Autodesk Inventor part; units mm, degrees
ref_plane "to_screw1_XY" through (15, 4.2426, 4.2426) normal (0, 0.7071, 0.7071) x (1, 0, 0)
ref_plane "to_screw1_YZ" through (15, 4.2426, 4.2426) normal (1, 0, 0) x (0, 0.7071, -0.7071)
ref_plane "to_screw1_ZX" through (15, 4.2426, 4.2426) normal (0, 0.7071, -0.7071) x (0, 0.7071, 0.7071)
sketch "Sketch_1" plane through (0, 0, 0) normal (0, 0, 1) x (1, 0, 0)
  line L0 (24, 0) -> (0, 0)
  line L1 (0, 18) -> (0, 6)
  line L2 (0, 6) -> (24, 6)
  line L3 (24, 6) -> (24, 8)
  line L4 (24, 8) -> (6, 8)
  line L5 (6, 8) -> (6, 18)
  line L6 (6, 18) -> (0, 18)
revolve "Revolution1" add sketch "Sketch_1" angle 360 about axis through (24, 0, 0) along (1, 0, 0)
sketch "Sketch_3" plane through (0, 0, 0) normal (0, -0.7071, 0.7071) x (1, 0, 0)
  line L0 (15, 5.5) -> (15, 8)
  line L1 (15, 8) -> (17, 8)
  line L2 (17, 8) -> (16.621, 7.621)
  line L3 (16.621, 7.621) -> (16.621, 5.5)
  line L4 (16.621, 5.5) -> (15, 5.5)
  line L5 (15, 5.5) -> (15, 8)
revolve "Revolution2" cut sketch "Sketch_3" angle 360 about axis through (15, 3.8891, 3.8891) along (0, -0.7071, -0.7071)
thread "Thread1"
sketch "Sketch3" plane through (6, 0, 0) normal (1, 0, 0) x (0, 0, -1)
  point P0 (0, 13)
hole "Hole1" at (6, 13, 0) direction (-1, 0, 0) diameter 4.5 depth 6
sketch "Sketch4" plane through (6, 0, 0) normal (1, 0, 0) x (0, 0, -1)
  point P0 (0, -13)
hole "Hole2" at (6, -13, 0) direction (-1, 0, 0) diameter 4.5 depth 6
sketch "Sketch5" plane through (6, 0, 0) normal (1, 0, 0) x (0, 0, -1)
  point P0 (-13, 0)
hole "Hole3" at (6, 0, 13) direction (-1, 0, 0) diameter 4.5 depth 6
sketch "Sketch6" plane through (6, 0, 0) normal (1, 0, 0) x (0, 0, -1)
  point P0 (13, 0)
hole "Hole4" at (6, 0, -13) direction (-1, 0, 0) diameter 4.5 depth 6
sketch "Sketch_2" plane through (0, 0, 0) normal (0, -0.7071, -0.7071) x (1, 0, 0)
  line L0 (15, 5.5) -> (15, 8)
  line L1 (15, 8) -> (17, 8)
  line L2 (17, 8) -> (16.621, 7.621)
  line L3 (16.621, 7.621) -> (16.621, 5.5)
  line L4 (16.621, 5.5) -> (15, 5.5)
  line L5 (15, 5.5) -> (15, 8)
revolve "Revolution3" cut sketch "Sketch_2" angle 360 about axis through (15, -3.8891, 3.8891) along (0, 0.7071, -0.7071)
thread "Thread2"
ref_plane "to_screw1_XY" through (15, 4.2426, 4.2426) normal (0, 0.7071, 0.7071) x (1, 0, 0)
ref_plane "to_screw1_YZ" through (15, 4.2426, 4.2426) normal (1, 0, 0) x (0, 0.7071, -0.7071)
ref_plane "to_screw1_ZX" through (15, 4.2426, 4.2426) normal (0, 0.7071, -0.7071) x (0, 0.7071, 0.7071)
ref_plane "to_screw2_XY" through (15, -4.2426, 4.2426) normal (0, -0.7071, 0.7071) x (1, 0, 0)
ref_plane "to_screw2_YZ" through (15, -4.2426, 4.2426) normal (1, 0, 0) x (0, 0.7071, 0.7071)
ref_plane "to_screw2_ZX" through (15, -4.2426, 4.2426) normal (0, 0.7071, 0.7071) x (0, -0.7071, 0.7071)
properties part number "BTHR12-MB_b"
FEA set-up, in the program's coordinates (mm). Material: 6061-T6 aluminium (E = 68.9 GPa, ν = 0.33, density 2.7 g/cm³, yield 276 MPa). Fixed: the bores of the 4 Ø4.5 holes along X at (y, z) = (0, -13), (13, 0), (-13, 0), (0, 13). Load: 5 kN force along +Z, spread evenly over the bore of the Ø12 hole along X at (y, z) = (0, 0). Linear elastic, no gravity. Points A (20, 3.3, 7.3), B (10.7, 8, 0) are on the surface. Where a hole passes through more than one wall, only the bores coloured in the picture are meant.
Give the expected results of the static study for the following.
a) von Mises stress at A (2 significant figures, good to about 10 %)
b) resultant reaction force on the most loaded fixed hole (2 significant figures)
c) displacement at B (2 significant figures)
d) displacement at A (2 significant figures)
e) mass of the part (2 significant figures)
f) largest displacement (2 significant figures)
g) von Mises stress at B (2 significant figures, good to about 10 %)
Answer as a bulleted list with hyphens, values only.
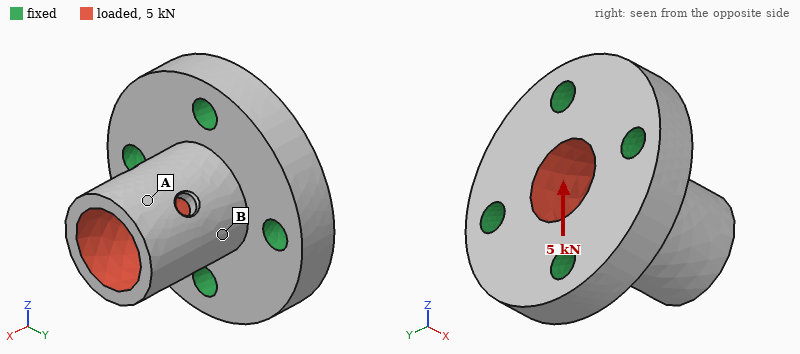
- 32 MPa
- 2.5 kN
- 22 µm
- 64 µm
- 18 g
- 77 µm
- 76 MPa
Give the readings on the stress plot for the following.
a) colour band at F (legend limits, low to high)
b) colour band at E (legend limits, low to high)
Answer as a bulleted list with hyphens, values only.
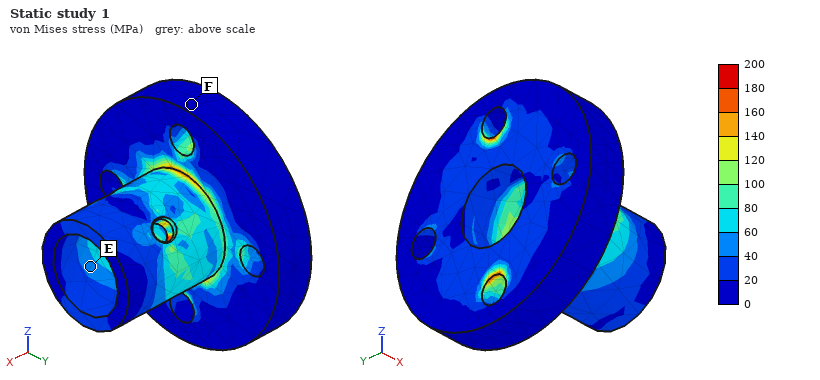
- 0 to 20 MPa
- 40 to 60 MPa
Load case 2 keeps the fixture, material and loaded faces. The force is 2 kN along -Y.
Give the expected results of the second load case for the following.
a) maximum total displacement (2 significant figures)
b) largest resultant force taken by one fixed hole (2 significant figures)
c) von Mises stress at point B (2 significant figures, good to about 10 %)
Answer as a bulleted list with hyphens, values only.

- 31 µm
- 990 N
- 24 MPa
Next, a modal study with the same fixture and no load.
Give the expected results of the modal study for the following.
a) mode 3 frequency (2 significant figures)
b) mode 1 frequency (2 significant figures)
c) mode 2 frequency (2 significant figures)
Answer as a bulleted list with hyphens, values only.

- 29 kHz
- 20 kHz
- 20 kHz
